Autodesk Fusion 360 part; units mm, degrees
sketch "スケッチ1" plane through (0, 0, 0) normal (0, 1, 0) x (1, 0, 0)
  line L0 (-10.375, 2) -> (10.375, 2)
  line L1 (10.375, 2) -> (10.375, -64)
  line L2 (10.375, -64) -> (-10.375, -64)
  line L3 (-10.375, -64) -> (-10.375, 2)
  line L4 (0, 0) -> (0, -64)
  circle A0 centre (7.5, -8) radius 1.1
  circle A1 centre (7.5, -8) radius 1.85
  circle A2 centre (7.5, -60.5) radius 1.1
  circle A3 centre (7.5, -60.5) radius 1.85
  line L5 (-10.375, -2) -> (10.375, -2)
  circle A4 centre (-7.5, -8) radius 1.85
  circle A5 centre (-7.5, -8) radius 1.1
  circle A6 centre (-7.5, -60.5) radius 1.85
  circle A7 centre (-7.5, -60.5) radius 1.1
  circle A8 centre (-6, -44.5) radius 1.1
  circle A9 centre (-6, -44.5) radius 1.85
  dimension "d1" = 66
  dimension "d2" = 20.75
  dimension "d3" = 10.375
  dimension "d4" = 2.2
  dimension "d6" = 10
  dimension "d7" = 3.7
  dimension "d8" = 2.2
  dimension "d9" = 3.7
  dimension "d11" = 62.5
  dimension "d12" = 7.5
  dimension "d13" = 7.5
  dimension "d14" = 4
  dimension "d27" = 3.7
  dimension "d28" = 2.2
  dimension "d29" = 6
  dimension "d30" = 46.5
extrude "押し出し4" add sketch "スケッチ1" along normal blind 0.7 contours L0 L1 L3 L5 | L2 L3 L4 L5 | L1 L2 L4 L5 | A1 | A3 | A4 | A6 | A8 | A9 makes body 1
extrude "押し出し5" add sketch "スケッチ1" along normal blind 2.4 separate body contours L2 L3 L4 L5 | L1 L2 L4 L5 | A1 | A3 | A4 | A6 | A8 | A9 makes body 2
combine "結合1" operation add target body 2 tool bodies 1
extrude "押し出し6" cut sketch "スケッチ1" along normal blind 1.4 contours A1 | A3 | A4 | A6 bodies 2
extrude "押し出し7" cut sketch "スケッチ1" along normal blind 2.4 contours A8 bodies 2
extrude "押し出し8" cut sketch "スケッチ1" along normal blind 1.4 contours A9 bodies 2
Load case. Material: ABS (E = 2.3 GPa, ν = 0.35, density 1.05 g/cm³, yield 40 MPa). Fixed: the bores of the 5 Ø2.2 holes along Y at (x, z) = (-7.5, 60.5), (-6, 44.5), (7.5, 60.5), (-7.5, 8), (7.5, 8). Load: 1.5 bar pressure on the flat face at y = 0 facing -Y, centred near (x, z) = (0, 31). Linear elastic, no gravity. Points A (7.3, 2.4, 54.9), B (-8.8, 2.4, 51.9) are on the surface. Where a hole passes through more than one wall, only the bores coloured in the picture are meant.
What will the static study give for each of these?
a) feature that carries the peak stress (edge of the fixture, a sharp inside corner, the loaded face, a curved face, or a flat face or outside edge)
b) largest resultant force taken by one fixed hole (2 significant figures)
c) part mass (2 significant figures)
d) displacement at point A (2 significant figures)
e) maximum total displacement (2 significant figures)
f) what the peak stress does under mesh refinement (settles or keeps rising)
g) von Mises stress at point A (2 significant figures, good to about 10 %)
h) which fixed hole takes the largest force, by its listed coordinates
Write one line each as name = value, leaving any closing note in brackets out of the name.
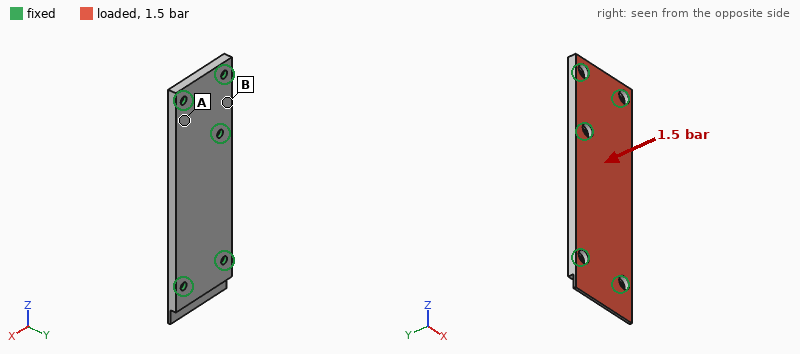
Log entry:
feature that carries the peak stress = edge of the fixture
largest resultant force taken by one fixed hole = 97 N
part mass = 3.2 g
displacement at point A = 0.13 mm
maximum total displacement = 0.81 mm
what the peak stress does under mesh refinement = keeps rising
von Mises stress at point A = 8.5 MPa
which fixed hole takes the largest force, by its listed coordinates = (-6, 44.5)
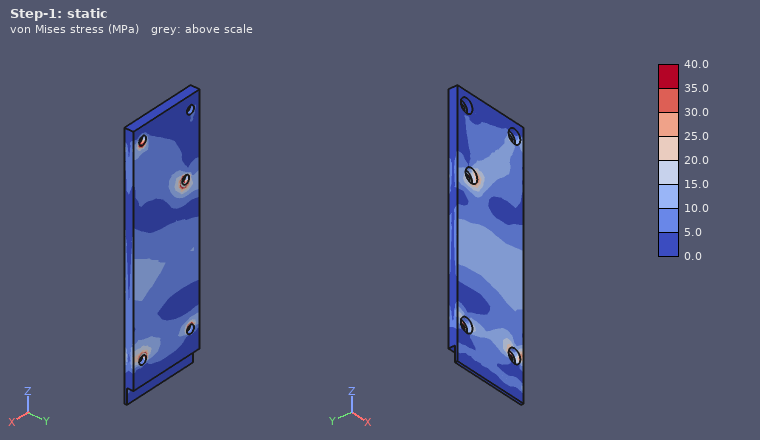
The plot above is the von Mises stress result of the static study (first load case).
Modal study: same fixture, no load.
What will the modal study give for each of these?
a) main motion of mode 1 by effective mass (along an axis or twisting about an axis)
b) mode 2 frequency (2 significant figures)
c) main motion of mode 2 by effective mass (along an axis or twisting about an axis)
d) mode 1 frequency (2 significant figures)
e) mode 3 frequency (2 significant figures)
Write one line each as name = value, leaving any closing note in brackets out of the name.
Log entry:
main motion of mode 1 by effective mass = along Y
mode 2 frequency = 2800 Hz
main motion of mode 2 by effective mass = twisting about Z
mode 1 frequency = 1700 Hz
mode 3 frequency = 4300 Hz
